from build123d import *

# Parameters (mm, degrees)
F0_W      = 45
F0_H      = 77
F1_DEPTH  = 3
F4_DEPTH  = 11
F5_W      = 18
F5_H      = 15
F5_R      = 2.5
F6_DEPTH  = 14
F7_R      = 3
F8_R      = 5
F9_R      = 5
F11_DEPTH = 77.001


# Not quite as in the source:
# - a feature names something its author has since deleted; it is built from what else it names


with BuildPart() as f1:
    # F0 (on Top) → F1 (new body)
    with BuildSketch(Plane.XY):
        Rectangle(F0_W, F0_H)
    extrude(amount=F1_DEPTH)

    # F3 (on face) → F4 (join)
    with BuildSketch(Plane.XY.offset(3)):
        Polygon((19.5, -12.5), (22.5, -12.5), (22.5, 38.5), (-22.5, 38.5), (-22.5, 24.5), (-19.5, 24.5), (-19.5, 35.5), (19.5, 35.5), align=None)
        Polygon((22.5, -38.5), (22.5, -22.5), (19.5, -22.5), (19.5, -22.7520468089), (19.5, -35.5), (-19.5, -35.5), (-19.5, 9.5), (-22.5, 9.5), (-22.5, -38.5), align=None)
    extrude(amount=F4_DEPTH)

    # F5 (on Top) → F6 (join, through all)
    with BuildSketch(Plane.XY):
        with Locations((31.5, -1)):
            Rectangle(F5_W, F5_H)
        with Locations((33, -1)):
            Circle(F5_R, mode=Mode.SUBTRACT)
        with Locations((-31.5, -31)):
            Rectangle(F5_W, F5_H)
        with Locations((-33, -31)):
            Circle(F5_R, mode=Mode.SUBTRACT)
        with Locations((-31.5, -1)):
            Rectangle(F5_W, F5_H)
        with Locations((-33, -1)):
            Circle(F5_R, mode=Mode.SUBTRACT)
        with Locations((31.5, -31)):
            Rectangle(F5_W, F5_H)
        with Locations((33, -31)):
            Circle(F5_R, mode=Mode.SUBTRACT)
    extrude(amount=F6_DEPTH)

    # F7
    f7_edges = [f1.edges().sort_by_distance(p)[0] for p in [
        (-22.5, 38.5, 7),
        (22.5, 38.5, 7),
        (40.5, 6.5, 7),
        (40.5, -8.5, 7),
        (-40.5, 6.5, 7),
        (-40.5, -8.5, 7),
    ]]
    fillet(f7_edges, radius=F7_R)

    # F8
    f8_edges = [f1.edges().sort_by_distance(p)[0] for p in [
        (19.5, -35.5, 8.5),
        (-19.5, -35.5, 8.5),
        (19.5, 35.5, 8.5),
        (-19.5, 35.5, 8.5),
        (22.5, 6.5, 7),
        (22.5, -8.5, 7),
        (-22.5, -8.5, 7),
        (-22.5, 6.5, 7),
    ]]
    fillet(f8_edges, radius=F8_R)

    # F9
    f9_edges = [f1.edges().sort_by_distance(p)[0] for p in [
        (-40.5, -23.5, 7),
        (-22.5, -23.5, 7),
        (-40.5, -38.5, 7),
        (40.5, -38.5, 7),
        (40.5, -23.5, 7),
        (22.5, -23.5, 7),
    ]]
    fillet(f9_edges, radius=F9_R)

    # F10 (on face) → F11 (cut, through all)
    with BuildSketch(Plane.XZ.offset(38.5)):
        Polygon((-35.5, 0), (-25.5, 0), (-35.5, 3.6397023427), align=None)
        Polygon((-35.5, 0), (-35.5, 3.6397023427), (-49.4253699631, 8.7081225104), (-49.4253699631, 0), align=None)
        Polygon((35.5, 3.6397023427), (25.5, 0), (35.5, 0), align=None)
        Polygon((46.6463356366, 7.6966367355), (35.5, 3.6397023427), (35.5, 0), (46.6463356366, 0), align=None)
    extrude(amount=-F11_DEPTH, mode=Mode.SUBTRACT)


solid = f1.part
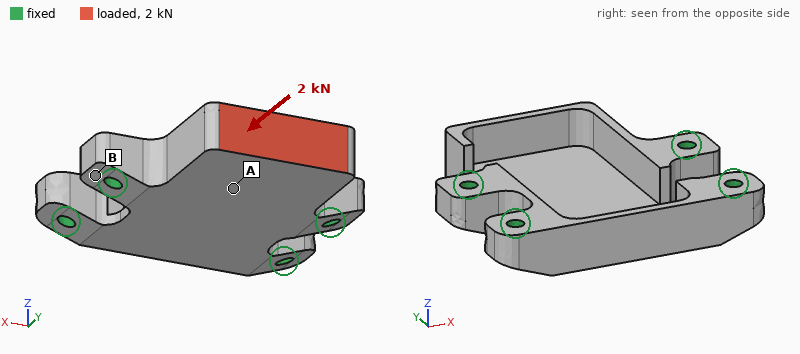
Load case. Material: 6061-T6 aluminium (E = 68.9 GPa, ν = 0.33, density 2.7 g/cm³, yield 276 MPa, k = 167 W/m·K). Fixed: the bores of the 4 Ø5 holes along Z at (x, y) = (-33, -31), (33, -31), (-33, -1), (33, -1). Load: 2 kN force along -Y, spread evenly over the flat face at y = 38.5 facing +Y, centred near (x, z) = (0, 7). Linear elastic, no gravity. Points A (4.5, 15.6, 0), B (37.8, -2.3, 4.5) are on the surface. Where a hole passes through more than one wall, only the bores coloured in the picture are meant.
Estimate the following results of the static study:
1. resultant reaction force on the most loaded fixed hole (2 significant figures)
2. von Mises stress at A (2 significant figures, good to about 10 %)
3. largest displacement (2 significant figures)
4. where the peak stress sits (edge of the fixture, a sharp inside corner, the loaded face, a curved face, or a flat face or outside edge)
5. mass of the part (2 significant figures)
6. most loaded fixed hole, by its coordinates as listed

870 N
19 MPa
0.37 mm
a curved face
79 g
(33, -1)
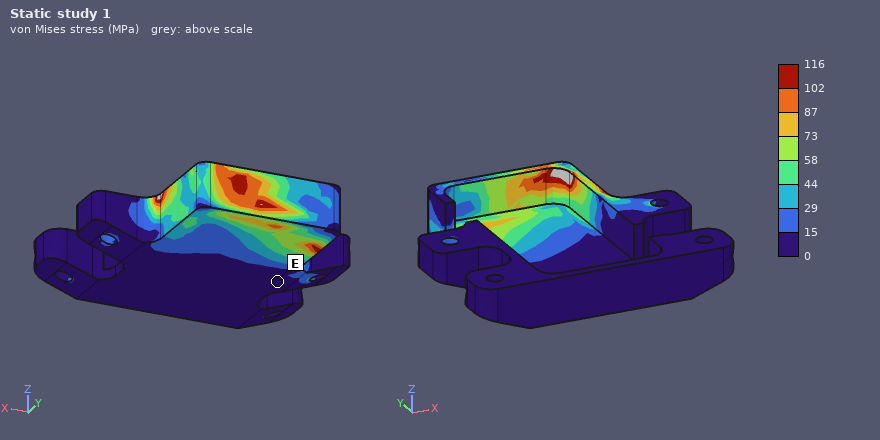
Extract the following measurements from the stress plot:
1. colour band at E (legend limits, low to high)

0 to 15 MPa
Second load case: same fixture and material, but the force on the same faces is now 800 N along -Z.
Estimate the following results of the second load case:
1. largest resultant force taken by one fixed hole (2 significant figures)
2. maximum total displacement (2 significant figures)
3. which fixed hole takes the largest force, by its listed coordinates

780 N
0.73 mm
(33, -1)
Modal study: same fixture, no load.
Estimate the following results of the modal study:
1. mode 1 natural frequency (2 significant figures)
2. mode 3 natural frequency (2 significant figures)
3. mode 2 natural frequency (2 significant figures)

2100 Hz
7700 Hz
4900 Hz
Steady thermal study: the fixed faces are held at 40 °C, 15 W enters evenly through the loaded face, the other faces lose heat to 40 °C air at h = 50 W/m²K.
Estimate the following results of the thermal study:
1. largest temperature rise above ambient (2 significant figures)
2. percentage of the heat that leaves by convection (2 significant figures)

22 K
22 %
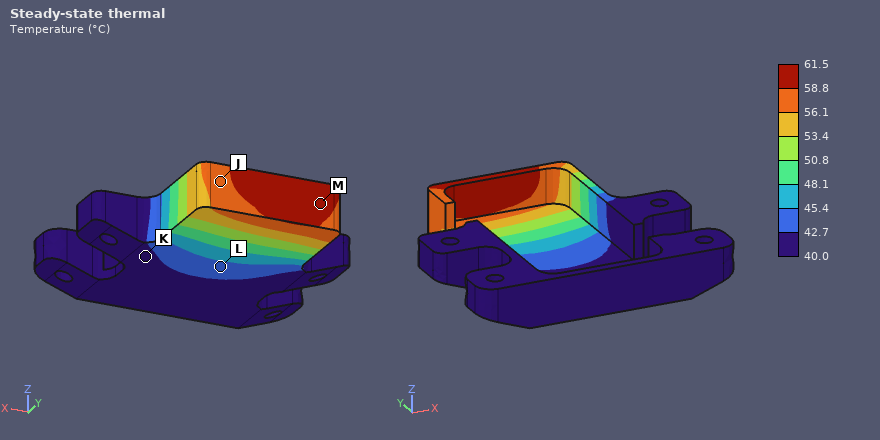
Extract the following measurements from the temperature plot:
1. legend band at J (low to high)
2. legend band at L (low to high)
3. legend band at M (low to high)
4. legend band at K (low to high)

56.1 to 58.8 °C
42.7 to 45.4 °C
58.8 to 61.5 °C
40.0 to 42.7 °C
